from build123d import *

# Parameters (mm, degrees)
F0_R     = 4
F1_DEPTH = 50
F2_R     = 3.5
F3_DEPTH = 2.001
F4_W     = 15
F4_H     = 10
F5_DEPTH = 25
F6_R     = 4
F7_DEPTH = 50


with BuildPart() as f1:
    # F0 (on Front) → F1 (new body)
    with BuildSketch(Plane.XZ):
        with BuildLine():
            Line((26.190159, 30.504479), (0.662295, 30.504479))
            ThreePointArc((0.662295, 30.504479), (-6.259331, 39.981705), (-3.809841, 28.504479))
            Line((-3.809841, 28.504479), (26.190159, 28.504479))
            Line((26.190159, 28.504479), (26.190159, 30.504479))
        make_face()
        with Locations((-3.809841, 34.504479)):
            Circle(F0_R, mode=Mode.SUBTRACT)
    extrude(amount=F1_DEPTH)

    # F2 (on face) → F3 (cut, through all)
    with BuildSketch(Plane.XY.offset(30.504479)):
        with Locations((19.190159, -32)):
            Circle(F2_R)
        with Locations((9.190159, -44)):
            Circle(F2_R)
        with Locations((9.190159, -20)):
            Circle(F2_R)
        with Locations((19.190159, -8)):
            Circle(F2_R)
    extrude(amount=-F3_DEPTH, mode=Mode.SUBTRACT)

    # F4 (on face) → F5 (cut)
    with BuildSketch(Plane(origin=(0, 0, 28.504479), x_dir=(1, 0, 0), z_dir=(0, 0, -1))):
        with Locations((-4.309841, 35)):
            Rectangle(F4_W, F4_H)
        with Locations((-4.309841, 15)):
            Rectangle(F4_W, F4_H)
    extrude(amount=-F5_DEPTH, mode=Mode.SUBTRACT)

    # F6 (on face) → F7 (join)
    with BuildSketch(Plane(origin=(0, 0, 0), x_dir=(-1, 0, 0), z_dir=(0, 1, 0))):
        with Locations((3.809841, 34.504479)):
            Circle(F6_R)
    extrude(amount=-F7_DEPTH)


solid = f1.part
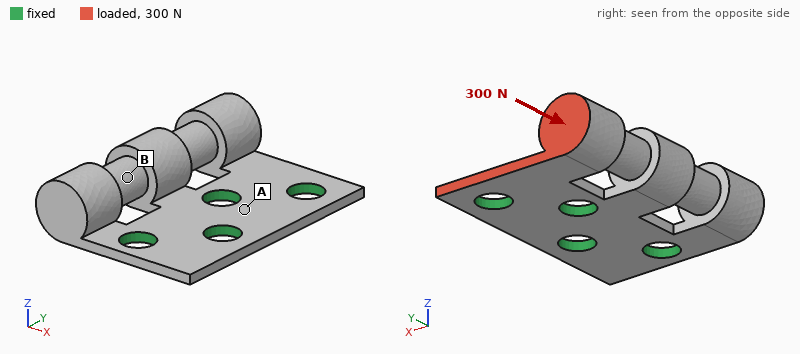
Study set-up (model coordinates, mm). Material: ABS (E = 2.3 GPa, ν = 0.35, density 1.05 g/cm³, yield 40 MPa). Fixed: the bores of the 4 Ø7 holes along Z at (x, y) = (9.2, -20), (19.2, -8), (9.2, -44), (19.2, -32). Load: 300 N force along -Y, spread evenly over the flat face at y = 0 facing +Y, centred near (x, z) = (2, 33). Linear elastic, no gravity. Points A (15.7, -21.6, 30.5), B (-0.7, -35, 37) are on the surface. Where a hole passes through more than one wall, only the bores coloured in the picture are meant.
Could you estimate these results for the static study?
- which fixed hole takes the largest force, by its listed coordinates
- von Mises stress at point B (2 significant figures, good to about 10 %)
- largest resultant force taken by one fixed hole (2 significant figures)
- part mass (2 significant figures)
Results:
(9.2, -20)
3.5 MPa
160 N
7.0 g
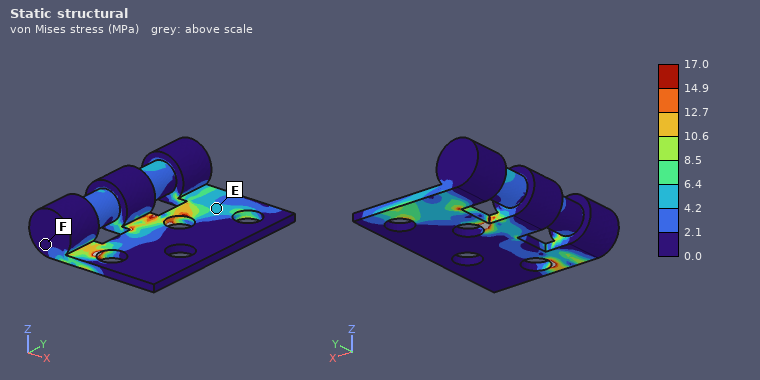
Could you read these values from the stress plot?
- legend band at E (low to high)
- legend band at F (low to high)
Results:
4.2 to 6.4 MPa
0.0 to 2.1 MPa
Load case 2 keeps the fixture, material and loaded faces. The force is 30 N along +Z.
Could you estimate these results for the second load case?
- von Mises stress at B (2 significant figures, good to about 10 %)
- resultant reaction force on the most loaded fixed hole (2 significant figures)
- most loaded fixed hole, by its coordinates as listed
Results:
3.0 MPa
42 N
(9.2, -20)
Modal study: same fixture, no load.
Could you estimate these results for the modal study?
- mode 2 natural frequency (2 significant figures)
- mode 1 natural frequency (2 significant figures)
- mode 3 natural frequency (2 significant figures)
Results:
1500 Hz
610 Hz
3100 Hz
